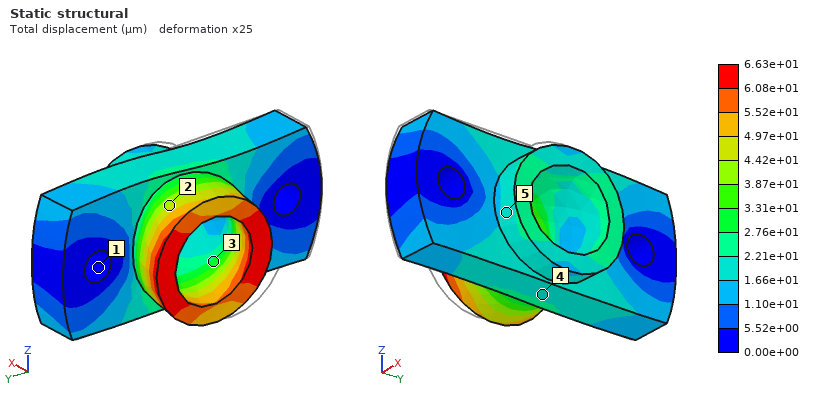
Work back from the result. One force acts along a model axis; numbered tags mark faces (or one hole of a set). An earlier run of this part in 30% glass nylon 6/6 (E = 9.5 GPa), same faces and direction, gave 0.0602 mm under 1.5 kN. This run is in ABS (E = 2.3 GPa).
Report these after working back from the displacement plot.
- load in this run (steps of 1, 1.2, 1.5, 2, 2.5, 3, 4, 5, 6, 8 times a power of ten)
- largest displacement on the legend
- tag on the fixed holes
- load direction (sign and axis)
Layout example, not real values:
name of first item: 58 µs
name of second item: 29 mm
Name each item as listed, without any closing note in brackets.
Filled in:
load in this run: 400 N
largest displacement on the legend: 6.63e+01 µm
tag on the fixed holes: 1
load direction: +Y
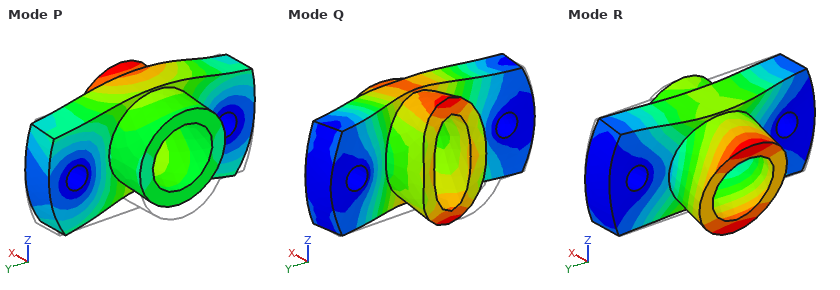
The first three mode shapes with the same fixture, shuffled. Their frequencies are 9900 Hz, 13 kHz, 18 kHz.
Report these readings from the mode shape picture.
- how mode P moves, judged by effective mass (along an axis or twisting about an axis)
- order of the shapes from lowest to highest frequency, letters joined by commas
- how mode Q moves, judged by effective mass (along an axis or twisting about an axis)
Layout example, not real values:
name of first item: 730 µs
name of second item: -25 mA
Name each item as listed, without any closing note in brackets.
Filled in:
how mode P moves, judged by effective mass: along Z
order of the shapes from lowest to highest frequency, letters joined by commas: R, Q, P
how mode Q moves, judged by effective mass: along X
